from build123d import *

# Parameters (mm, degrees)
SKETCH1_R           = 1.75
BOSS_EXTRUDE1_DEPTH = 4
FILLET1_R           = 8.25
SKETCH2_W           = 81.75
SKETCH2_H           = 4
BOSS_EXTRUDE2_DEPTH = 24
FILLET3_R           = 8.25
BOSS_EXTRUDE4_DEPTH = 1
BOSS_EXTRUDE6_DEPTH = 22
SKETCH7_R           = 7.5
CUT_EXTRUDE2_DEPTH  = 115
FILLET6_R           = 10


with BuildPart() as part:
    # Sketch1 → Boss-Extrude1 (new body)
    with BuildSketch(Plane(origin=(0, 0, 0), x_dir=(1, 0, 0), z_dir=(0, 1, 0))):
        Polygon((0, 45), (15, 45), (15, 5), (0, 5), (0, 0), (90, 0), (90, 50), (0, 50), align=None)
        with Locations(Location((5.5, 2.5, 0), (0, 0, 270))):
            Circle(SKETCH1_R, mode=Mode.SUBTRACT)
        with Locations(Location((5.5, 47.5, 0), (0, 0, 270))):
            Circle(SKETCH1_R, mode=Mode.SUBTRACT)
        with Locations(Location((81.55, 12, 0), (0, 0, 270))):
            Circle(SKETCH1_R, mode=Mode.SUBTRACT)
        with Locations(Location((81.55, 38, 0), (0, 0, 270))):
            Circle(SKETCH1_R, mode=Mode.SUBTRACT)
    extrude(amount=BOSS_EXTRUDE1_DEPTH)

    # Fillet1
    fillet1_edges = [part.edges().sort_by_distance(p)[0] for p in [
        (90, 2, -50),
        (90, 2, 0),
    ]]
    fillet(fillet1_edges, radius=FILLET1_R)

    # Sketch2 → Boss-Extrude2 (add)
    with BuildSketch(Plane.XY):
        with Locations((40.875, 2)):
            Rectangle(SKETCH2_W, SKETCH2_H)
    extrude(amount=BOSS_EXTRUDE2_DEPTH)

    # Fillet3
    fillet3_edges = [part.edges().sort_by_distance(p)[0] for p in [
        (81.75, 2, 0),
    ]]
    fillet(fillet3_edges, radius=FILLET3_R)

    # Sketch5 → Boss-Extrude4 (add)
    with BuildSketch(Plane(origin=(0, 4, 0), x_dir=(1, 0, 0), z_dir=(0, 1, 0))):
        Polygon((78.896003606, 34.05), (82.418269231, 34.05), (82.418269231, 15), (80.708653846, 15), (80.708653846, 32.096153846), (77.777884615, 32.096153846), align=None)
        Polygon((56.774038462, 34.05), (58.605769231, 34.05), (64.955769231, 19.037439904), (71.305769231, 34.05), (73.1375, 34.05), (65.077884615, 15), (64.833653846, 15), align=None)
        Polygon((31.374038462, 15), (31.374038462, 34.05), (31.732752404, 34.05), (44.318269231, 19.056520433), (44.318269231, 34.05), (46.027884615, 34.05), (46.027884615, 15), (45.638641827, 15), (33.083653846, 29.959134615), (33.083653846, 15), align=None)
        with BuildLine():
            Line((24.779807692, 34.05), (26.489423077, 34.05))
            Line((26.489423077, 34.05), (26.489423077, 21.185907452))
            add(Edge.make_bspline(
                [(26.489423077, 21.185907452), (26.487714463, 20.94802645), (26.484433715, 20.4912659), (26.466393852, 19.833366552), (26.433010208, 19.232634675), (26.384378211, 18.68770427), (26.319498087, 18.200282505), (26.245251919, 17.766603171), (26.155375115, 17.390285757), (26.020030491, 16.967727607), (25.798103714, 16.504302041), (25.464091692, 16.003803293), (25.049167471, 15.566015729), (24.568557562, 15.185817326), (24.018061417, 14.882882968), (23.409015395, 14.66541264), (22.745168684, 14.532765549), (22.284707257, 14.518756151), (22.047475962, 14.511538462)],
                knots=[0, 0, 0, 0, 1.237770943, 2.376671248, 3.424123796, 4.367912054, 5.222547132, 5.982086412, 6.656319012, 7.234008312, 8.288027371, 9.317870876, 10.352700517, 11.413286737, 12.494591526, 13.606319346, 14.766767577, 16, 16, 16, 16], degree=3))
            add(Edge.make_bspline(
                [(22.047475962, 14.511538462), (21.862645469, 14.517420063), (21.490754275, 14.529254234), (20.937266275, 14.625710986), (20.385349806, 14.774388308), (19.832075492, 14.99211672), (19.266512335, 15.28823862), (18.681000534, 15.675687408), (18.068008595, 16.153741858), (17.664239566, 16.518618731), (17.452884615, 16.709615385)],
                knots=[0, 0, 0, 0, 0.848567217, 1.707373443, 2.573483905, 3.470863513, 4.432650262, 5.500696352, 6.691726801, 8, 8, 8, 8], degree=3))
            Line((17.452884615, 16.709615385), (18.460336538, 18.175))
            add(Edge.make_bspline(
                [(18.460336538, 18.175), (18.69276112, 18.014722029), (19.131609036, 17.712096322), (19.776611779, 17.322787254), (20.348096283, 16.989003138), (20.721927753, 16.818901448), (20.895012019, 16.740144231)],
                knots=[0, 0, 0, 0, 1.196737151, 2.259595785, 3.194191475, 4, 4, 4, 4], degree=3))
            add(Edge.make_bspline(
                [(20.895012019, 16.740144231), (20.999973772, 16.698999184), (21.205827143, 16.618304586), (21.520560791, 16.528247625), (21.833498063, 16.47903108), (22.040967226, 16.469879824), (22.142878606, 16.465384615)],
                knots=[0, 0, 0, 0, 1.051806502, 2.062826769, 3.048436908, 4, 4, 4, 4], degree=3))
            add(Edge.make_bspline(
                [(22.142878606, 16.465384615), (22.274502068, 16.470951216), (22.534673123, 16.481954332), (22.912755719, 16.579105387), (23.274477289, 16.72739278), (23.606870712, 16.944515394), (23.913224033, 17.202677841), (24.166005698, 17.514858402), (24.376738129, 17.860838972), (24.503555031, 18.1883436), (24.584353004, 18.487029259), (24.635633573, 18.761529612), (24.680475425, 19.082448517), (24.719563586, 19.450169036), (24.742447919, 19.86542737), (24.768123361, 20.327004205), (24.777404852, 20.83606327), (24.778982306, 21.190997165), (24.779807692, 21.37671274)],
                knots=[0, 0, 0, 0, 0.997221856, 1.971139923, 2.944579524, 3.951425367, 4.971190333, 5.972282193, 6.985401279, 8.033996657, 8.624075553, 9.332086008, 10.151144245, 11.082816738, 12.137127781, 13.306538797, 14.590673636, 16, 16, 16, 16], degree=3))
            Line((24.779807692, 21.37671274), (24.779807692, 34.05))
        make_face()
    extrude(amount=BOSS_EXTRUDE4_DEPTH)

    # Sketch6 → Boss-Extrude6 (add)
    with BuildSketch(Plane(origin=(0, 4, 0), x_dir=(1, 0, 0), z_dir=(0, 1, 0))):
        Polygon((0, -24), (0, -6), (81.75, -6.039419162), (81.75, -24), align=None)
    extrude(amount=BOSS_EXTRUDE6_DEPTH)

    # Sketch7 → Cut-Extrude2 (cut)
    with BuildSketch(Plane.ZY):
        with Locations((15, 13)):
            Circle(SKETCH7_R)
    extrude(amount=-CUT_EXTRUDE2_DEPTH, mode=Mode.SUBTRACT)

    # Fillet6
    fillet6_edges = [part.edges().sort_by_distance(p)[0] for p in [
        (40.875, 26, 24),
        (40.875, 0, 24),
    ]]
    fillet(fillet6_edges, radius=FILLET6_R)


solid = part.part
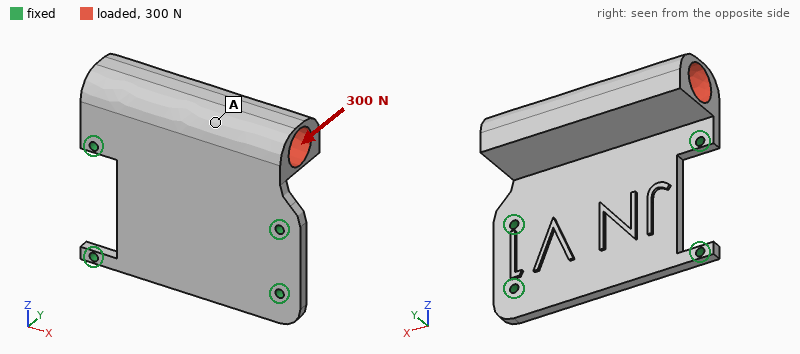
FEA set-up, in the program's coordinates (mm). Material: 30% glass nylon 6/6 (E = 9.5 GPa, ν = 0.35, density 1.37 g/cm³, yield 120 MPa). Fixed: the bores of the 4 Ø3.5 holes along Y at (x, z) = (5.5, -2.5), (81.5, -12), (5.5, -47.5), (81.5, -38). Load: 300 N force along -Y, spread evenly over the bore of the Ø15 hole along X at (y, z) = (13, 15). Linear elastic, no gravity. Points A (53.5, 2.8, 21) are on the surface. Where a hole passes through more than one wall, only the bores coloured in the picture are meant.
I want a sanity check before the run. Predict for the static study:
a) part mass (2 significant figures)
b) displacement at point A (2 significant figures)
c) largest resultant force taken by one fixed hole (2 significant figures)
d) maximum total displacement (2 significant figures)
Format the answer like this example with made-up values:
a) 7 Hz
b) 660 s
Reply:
a) 52 g
b) 0.55 mm
c) 200 N
d) 0.76 mm
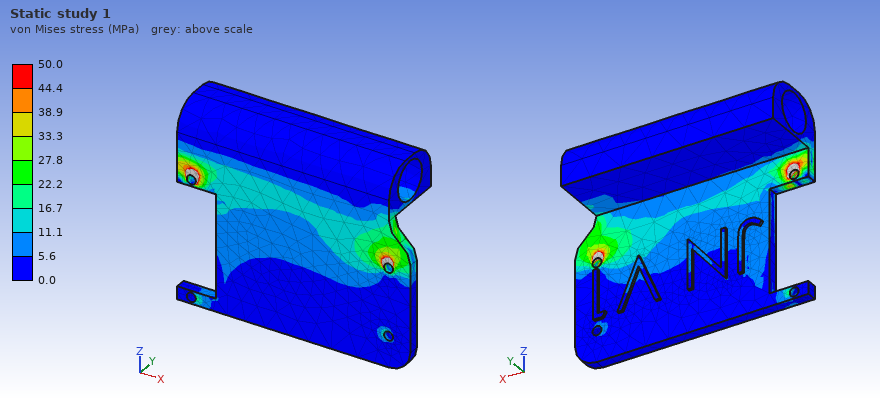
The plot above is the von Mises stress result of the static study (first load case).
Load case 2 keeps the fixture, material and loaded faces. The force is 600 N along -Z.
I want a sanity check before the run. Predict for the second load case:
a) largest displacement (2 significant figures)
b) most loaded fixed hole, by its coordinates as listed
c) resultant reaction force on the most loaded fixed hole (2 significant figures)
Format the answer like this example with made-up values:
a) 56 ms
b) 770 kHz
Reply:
a) 0.95 mm
b) (5.5, -2.5)
c) 270 N
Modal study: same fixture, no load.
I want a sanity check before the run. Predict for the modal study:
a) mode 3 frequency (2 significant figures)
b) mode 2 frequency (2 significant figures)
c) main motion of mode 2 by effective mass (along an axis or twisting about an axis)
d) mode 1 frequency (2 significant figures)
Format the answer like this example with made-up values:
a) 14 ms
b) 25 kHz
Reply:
a) 2000 Hz
b) 1700 Hz
c) along Y
d) 660 Hz
